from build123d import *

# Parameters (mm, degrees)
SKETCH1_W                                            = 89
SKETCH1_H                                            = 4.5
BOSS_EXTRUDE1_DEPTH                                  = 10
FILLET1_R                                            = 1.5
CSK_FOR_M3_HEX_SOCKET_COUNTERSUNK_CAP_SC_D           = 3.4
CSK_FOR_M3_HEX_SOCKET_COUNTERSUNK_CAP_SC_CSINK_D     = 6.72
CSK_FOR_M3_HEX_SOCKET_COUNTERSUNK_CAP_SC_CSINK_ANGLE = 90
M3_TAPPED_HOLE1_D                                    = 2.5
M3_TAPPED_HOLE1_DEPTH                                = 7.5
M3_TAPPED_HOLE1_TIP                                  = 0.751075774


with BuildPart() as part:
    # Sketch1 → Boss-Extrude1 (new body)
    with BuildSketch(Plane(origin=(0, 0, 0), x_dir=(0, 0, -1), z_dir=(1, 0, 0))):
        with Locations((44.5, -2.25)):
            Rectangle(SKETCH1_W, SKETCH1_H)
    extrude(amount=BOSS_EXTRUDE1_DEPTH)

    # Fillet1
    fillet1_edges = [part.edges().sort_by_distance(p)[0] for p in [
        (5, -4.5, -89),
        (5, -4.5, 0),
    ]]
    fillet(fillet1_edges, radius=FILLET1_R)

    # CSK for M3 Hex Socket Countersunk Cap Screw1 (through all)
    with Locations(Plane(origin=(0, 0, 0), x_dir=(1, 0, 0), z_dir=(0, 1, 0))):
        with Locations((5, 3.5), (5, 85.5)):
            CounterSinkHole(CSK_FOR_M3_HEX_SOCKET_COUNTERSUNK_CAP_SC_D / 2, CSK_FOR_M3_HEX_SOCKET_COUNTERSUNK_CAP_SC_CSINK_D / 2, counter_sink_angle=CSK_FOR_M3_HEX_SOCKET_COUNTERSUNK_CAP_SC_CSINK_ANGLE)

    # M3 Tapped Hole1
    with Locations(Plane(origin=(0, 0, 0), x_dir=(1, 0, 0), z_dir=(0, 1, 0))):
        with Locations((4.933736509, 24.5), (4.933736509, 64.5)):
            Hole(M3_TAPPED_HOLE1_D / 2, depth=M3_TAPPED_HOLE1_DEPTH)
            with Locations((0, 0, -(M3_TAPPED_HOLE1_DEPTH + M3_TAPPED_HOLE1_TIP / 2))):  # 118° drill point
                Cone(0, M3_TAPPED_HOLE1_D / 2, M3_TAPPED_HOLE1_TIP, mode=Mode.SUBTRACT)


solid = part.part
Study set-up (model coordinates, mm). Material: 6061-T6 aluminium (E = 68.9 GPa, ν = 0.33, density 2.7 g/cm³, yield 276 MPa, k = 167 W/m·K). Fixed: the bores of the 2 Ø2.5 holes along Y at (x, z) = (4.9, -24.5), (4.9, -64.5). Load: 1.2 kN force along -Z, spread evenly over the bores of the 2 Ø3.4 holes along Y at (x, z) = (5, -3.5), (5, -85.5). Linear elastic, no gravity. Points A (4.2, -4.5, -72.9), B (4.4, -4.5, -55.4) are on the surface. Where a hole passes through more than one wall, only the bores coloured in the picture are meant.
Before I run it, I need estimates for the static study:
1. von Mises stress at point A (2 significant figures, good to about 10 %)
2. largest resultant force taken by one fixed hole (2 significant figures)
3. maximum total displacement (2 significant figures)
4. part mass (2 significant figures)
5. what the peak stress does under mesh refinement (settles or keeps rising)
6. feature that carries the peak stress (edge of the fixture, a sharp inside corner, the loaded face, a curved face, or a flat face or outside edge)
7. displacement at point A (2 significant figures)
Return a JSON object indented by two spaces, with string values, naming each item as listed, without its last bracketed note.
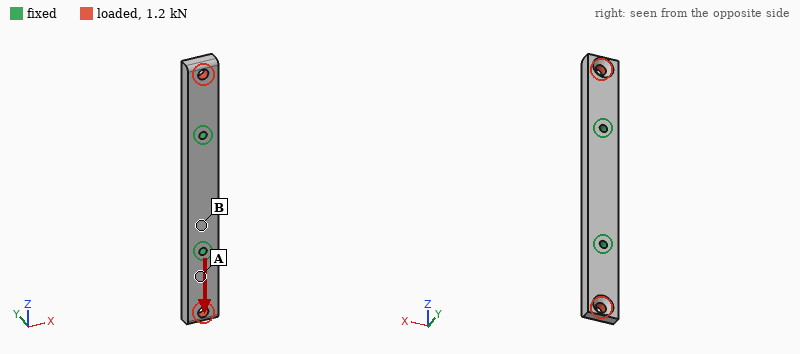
{
  "von Mises stress at point A": "29 MPa",
  "largest resultant force taken by one fixed hole": "600 N",
  "maximum total displacement": "29 µm",
  "part mass": "10 g",
  "what the peak stress does under mesh refinement": "keeps rising",
  "feature that carries the peak stress": "edge of the fixture",
  "displacement at point A": "5.2 µm"
}
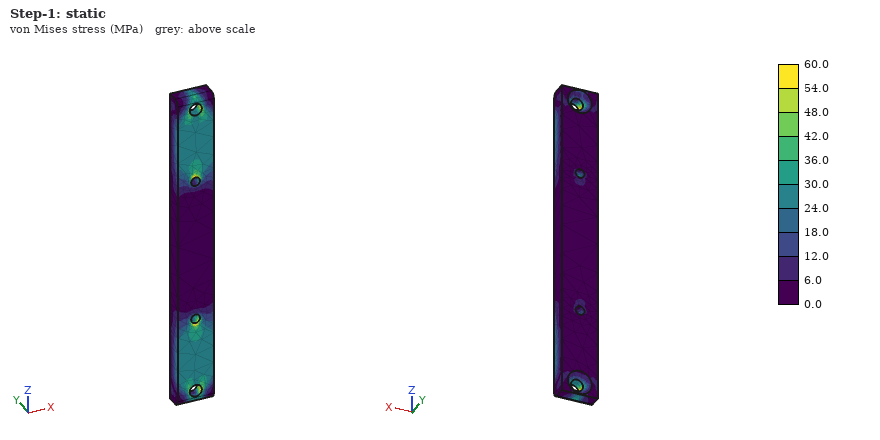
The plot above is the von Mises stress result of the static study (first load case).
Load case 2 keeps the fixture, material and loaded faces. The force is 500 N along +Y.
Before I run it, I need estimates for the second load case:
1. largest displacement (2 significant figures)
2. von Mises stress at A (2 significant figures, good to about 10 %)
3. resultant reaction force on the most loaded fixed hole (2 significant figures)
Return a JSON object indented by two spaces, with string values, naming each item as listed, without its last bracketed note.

{
  "largest displacement": "0.20 mm",
  "von Mises stress at A": "92 MPa",
  "resultant reaction force on the most loaded fixed hole": "250 N"
}
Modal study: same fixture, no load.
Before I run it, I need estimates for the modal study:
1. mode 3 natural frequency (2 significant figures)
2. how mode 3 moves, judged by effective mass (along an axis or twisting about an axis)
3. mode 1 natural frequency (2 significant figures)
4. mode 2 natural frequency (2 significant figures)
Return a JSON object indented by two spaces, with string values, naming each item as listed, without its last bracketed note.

{
  "mode 3 natural frequency": "9300 Hz",
  "how mode 3 moves, judged by effective mass": "along X",
  "mode 1 natural frequency": "6400 Hz",
  "mode 2 natural frequency": "6500 Hz"
}
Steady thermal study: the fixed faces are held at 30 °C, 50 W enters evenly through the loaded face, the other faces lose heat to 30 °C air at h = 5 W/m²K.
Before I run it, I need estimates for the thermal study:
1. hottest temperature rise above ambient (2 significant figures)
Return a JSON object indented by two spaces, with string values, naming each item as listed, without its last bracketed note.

{
  "hottest temperature rise above ambient": "82 K"
}
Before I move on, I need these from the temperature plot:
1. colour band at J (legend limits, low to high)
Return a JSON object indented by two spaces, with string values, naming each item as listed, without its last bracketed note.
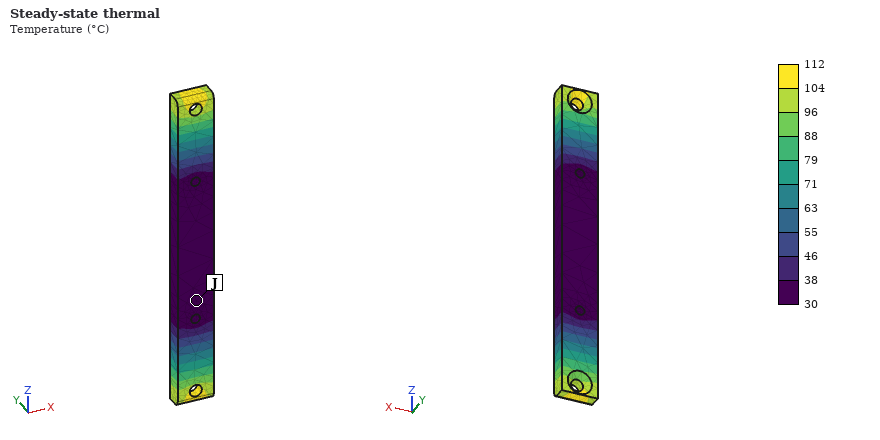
{
  "colour band at J": "30 to 38 °C"
}
